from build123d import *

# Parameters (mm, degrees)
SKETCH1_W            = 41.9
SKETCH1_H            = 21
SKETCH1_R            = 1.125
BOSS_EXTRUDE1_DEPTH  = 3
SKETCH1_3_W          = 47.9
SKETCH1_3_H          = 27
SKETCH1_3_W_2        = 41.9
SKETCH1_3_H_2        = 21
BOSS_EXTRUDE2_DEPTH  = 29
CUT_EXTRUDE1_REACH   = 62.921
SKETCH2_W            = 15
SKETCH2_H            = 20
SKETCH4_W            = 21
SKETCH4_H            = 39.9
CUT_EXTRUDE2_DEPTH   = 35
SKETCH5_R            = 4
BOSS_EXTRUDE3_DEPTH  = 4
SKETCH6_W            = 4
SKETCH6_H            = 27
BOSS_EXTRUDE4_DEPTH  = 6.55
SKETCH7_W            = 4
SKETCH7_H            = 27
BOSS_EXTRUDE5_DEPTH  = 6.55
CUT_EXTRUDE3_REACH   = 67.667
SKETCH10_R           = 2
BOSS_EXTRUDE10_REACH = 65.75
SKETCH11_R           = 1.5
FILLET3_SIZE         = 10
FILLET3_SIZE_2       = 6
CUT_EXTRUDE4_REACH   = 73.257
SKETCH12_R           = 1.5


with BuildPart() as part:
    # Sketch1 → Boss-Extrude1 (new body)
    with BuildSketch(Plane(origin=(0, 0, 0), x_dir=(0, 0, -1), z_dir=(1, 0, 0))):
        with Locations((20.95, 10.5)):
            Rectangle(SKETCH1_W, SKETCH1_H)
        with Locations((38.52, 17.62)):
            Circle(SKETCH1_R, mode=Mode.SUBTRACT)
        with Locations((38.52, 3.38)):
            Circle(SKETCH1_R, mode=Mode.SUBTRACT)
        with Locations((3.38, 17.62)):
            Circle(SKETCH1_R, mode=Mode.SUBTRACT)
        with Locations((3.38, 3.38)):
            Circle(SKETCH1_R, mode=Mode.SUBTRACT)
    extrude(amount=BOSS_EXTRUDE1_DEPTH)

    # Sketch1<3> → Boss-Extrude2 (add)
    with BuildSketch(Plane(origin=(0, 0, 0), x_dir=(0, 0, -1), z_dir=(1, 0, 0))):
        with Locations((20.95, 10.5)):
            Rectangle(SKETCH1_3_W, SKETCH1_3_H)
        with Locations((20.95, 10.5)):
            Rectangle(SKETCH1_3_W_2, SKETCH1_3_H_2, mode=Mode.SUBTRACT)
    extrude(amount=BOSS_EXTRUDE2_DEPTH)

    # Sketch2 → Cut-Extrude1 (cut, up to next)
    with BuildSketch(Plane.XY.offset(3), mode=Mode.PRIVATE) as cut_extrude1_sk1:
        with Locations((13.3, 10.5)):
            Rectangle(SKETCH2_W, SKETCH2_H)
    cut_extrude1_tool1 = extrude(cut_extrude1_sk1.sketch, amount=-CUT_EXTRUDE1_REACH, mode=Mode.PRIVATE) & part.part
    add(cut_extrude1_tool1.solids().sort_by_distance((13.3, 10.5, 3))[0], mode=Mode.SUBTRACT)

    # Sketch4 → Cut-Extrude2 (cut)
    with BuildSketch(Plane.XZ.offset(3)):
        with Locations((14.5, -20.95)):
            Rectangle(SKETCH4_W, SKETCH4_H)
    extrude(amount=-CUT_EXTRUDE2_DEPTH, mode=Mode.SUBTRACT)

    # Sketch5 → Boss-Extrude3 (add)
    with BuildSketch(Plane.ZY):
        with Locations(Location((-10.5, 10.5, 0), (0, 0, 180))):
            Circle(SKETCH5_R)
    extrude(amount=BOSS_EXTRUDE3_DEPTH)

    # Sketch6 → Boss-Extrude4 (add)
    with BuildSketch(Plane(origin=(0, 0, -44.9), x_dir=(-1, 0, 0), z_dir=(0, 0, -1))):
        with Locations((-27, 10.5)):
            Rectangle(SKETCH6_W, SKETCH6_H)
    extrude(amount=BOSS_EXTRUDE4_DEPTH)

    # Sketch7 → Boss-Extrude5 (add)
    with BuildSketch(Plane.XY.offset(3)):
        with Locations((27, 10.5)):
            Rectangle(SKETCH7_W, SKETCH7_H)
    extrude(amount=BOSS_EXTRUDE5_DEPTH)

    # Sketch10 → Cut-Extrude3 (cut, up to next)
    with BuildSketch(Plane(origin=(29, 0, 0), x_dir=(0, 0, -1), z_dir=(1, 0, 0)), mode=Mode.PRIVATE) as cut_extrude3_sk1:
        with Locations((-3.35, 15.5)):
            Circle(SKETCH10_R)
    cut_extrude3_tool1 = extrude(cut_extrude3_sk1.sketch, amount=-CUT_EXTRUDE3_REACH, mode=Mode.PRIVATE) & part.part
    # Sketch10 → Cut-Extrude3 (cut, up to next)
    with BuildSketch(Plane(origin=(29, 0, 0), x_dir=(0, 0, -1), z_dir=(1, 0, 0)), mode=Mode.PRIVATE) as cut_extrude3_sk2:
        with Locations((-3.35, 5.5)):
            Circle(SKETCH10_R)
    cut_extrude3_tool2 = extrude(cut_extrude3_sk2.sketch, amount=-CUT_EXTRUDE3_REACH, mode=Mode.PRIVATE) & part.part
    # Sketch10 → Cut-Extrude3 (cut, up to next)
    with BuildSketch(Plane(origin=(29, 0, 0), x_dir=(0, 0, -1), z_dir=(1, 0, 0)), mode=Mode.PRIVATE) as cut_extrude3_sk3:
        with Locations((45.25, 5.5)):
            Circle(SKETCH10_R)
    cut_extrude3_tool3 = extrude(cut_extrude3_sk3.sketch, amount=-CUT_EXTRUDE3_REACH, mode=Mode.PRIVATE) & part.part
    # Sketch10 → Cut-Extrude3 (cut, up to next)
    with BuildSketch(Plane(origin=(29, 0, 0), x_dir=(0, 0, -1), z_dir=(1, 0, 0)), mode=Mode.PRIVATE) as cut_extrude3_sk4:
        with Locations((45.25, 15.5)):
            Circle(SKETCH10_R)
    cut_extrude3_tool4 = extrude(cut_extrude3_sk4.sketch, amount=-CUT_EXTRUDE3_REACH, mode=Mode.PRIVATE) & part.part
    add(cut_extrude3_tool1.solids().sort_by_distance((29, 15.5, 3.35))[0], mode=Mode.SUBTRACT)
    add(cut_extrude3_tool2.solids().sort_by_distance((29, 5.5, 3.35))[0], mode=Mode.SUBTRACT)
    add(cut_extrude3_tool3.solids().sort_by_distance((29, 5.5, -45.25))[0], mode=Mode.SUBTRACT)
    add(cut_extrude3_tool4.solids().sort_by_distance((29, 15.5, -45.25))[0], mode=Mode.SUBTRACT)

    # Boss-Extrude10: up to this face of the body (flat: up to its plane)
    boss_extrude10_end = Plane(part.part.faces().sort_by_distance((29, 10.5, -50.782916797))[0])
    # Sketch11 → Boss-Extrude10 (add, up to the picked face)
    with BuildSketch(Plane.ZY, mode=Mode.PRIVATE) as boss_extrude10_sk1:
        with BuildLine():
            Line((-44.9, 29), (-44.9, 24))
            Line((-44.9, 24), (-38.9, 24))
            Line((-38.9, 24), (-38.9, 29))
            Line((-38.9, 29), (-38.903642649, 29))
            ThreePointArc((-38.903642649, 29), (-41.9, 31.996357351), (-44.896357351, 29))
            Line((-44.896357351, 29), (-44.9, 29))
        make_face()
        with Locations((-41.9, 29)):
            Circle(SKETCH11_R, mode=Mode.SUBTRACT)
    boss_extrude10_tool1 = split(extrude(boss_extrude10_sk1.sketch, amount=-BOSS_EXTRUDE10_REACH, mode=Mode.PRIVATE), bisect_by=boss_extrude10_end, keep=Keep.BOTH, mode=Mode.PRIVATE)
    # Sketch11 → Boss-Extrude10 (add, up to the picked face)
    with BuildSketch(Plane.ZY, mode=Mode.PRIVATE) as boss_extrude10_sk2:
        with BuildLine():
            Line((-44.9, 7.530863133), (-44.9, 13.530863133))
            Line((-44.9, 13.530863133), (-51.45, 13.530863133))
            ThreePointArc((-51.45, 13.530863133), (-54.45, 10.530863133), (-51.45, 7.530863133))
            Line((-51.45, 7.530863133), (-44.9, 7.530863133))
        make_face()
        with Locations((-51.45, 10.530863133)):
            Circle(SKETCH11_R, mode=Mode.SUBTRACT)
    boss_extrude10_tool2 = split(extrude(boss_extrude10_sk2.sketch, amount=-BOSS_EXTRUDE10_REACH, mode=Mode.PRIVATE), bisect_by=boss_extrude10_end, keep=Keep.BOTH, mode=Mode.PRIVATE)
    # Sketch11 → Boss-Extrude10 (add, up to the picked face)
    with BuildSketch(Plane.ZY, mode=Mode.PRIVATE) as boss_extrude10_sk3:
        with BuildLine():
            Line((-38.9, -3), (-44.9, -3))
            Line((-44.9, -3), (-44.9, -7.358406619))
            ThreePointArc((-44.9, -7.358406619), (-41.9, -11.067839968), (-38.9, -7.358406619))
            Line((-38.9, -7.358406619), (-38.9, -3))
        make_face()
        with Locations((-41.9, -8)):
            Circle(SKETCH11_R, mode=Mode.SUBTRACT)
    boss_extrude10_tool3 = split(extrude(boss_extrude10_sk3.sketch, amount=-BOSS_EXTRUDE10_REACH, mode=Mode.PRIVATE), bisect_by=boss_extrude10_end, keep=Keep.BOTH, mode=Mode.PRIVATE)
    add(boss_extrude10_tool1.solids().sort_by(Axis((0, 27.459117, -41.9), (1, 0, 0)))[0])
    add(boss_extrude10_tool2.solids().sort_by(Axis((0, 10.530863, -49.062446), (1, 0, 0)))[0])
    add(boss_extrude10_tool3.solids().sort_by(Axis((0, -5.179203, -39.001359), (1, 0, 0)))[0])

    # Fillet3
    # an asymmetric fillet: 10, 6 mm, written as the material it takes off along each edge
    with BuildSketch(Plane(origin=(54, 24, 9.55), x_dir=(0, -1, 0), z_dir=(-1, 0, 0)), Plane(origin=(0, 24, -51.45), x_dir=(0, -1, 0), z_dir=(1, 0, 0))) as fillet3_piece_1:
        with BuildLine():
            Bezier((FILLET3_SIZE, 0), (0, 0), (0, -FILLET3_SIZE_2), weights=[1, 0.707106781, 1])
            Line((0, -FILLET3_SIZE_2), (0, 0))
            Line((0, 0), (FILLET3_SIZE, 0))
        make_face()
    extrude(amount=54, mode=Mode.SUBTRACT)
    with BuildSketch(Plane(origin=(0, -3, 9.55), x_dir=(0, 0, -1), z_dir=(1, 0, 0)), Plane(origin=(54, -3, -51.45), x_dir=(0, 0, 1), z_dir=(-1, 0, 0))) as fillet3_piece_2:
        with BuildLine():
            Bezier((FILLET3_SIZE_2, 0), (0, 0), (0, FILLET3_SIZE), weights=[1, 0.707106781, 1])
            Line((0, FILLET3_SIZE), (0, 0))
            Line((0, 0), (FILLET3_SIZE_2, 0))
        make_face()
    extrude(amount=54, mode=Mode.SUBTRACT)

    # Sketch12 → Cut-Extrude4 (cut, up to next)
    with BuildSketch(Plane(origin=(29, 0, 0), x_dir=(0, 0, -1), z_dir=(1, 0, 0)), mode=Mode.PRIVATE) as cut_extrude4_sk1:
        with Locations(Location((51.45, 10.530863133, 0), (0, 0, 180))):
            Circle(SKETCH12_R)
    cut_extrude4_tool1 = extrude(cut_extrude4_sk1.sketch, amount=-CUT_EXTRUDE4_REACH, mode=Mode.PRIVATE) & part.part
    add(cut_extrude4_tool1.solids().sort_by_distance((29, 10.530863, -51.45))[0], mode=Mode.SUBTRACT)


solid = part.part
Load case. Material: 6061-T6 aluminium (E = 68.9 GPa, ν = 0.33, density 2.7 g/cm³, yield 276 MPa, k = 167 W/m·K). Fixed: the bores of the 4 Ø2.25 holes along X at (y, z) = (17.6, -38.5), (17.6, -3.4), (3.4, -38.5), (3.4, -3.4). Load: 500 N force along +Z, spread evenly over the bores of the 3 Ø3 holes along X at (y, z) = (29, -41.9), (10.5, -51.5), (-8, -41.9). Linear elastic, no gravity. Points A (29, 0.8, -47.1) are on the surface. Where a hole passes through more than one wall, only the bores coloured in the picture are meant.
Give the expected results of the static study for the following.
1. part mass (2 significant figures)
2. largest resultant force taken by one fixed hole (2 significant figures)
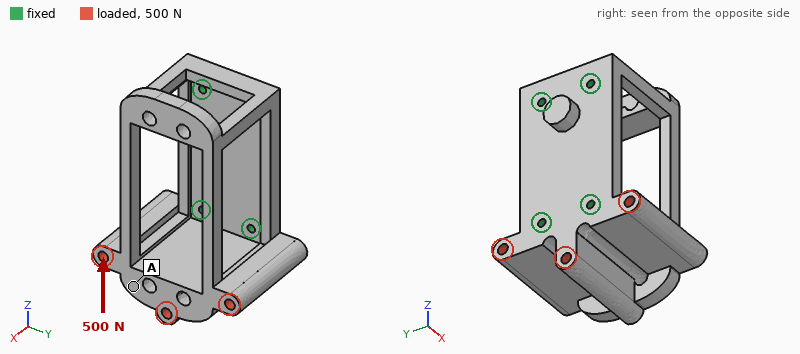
35 g
170 N
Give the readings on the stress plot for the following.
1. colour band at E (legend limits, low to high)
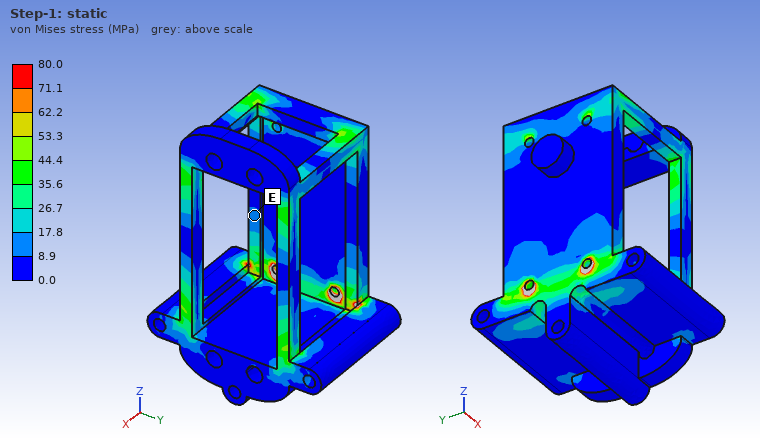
8.9 to 17.8 MPa
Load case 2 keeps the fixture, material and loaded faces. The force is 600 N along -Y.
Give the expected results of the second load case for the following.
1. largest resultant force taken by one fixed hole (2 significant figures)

580 N
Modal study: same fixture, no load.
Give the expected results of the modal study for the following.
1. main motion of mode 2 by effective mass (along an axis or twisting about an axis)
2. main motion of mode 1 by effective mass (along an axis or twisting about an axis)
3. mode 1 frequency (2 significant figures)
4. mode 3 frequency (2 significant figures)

along Y
along Z
2400 Hz
5000 Hz
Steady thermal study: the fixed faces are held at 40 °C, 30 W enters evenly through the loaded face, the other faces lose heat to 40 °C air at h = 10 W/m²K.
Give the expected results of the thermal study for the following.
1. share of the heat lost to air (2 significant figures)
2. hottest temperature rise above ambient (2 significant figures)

3.6 %
24 K
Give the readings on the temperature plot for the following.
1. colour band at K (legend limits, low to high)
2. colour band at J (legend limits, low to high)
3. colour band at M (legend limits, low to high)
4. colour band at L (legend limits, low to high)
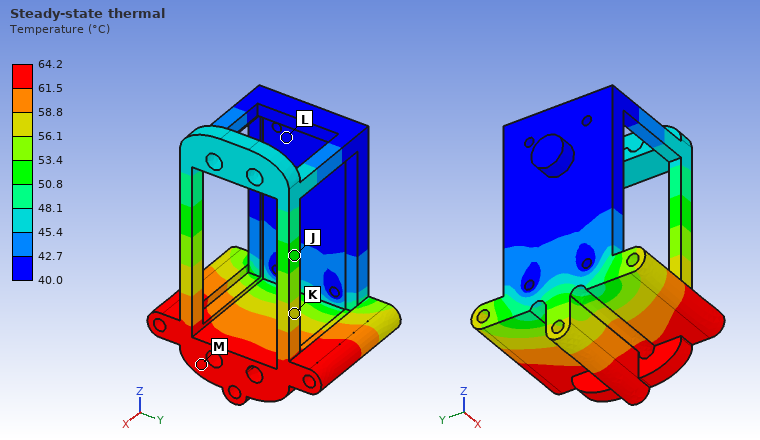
56.1 to 58.8 °C
50.8 to 53.4 °C
61.5 to 64.2 °C
40.0 to 42.7 °C
